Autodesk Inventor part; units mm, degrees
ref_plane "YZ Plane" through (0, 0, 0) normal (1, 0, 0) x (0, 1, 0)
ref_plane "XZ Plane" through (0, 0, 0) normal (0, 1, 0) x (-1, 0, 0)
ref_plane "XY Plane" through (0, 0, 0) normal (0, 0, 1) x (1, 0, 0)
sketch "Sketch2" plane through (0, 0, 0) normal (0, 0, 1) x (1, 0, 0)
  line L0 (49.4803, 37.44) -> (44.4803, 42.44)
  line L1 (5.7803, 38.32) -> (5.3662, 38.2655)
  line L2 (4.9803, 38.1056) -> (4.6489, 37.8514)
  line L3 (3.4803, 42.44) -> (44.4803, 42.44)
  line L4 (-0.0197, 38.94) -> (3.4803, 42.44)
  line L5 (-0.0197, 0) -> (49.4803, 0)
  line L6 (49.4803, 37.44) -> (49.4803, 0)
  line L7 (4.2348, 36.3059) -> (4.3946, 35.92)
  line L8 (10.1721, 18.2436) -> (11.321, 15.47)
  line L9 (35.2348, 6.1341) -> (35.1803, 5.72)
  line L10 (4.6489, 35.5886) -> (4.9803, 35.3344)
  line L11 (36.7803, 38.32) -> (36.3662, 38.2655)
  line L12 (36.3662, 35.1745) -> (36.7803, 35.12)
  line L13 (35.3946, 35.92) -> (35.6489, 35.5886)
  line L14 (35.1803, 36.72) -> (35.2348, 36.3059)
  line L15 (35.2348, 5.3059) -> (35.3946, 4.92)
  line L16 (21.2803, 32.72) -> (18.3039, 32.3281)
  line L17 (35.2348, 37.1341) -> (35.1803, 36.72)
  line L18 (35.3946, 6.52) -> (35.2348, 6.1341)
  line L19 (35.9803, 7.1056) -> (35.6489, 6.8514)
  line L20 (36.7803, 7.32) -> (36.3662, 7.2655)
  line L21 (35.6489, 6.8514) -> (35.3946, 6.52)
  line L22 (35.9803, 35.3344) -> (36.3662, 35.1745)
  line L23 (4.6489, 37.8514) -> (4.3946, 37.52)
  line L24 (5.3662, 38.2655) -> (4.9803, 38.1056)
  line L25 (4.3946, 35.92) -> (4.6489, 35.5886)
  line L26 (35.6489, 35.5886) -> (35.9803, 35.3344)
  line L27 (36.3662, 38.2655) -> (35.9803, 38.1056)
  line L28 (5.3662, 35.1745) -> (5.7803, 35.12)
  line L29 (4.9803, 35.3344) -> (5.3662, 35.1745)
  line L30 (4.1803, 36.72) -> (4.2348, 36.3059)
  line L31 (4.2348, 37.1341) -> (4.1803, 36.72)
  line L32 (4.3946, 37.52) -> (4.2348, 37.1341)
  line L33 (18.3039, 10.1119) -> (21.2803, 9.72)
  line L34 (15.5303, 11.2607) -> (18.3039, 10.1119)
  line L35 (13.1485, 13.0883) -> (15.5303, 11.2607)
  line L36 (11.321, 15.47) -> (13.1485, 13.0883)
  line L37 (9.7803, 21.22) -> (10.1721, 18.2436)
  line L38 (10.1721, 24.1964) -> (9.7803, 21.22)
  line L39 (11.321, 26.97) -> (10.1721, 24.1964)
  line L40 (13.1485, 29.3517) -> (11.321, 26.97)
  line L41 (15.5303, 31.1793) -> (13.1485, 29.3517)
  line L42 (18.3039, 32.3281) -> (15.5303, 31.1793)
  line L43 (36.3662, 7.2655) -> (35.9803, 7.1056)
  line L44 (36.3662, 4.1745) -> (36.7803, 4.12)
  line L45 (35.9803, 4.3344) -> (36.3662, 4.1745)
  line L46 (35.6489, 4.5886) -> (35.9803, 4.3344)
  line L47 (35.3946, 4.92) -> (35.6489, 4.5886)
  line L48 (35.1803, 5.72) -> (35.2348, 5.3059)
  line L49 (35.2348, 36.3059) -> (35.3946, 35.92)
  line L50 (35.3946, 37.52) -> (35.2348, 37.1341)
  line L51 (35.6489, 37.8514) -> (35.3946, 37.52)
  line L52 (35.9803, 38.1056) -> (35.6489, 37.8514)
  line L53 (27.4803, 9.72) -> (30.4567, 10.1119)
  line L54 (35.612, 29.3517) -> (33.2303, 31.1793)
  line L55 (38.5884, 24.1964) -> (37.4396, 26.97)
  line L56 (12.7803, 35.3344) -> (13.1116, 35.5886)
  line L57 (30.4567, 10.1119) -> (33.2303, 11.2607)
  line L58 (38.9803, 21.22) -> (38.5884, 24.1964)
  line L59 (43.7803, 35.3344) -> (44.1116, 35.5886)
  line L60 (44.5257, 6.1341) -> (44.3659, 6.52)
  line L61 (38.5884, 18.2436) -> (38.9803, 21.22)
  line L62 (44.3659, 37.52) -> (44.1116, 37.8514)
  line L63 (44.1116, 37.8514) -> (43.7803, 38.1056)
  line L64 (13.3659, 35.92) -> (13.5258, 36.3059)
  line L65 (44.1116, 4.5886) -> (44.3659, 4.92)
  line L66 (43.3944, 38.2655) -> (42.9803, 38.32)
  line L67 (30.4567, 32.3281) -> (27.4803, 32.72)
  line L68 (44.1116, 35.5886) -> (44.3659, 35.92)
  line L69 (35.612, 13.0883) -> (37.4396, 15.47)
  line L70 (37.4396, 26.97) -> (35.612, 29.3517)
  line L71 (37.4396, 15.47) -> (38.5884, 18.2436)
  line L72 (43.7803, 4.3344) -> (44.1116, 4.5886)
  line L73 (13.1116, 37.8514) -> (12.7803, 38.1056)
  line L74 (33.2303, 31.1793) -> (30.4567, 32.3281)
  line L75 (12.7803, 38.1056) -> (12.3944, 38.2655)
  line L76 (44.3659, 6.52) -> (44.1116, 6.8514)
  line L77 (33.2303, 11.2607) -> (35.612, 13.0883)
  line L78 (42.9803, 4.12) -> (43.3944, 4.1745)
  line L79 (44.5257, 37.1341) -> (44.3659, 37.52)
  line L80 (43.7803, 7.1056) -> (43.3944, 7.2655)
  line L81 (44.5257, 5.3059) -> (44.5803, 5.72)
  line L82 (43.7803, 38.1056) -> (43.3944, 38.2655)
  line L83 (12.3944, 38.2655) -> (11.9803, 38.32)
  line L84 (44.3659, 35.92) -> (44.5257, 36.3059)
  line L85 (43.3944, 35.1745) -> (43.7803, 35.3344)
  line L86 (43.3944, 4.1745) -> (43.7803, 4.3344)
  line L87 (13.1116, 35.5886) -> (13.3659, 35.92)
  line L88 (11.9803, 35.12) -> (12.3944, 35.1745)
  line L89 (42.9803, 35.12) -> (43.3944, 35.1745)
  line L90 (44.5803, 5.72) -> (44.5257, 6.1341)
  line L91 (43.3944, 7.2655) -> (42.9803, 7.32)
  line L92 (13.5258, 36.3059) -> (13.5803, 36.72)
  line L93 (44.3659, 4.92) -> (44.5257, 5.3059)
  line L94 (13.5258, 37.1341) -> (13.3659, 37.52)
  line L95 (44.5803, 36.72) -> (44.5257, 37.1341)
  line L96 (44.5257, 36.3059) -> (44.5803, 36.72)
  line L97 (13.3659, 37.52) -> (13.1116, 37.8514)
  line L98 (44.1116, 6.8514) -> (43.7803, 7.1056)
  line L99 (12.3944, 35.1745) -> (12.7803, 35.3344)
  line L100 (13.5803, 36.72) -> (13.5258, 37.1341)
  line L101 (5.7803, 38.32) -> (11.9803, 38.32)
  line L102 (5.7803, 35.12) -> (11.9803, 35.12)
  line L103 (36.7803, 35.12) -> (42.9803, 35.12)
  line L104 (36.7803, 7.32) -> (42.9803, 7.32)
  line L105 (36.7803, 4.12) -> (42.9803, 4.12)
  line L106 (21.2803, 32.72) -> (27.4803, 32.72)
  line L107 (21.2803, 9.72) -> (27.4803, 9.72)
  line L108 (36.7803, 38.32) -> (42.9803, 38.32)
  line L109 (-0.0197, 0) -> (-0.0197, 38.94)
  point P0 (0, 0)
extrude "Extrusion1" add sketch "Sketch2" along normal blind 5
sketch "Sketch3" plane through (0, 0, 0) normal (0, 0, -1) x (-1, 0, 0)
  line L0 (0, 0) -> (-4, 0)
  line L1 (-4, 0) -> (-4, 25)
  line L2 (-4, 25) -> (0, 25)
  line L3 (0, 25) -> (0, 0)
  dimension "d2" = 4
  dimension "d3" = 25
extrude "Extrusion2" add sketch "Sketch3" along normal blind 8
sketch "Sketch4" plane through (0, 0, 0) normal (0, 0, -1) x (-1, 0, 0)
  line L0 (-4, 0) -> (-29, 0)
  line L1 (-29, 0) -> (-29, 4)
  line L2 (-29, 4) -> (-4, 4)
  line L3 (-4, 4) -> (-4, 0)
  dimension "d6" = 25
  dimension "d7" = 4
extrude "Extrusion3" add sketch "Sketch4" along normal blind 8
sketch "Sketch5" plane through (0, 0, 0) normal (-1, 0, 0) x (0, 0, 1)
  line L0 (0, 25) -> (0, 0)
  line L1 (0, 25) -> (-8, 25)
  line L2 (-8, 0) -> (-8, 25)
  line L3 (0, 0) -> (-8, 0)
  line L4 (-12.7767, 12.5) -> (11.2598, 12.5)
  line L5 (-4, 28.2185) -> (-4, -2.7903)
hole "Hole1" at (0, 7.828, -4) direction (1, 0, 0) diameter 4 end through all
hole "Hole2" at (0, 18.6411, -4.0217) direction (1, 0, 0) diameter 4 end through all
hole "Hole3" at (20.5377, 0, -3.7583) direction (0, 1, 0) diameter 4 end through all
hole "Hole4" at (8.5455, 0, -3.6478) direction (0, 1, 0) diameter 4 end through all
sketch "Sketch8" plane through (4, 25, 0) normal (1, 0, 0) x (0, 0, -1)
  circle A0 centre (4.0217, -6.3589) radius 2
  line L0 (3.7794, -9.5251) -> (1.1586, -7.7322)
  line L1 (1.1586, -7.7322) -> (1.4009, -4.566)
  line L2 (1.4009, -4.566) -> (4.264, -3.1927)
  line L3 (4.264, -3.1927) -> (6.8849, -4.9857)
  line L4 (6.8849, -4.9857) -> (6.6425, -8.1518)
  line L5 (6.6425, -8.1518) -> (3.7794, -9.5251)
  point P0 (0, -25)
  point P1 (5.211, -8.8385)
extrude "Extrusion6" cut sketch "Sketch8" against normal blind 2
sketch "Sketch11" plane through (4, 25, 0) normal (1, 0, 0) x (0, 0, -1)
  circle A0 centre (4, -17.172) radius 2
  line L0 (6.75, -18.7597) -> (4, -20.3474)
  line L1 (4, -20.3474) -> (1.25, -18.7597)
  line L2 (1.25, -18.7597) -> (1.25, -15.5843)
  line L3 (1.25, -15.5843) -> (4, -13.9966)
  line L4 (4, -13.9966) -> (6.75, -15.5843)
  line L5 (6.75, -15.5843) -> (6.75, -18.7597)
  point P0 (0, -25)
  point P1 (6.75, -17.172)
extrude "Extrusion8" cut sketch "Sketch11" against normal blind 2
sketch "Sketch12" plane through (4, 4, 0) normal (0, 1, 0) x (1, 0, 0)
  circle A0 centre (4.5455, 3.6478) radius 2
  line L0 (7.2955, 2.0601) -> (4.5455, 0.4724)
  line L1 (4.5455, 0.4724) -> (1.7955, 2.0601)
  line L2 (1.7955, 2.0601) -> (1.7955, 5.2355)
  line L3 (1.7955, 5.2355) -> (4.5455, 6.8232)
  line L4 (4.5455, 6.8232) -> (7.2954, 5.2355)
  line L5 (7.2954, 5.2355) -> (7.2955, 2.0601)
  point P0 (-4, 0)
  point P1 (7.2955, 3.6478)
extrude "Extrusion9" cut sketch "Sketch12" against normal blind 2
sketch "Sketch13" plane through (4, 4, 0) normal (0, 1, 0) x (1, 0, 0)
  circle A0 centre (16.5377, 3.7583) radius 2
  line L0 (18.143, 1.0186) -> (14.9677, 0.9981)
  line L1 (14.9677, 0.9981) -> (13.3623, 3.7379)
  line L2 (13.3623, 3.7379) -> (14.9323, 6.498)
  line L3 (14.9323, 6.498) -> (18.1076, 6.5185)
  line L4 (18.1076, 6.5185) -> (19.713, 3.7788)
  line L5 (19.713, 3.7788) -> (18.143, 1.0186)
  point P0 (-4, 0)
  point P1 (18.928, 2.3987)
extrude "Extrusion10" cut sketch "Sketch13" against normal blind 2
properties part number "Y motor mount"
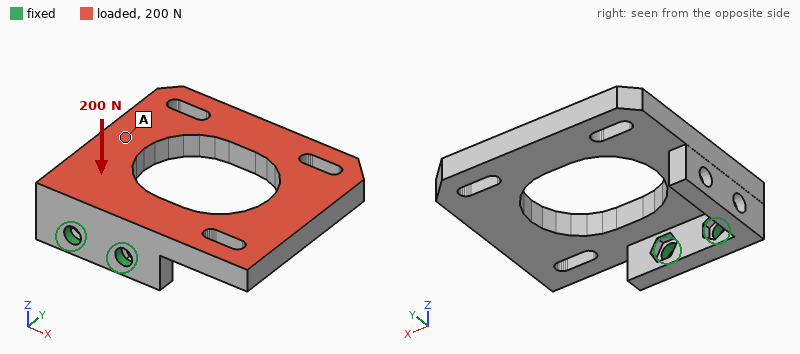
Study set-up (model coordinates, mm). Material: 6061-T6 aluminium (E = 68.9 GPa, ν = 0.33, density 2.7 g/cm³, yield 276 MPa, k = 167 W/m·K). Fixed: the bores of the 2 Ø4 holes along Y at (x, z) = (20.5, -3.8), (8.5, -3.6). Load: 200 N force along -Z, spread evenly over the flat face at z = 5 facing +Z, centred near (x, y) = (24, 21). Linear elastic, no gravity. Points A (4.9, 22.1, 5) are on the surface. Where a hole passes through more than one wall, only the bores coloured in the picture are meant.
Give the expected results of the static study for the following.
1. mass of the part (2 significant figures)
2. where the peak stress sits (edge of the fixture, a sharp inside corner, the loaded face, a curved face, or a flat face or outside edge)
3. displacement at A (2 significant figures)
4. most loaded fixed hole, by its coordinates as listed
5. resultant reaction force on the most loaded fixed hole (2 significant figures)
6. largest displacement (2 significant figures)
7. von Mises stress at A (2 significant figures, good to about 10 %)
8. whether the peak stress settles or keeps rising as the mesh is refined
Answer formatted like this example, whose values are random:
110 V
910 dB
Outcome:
23 g
edge of the fixture
0.068 mm
(20.5, -3.8)
250 N
0.25 mm
23 MPa
keeps rising
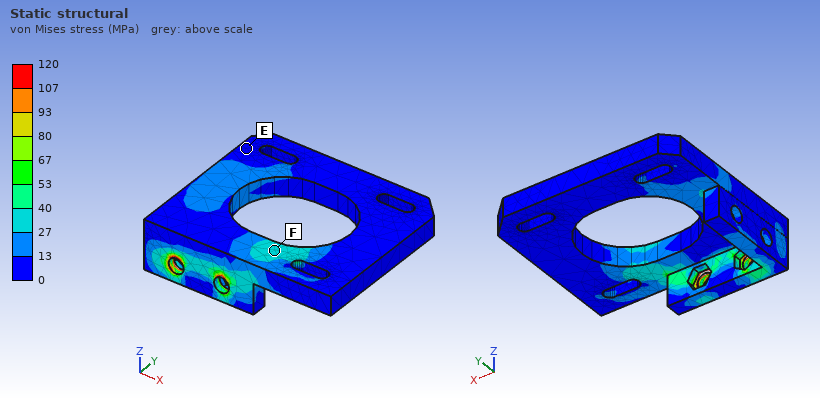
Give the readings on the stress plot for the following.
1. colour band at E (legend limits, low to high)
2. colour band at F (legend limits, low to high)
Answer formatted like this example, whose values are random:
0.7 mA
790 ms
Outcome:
0 to 13 MPa
27 to 40 MPa
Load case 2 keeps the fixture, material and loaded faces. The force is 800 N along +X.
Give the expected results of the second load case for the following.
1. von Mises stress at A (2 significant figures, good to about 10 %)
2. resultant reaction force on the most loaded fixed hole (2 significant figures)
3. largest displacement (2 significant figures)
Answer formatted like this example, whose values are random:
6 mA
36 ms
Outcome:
17 MPa
1.3 kN
0.15 mm
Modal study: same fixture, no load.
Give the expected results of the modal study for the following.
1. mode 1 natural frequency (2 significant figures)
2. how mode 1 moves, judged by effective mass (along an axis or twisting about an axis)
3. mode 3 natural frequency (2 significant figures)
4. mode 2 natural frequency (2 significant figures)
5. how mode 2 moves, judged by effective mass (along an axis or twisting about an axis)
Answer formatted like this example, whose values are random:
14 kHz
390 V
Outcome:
1300 Hz
along Z
3300 Hz
2400 Hz
along X
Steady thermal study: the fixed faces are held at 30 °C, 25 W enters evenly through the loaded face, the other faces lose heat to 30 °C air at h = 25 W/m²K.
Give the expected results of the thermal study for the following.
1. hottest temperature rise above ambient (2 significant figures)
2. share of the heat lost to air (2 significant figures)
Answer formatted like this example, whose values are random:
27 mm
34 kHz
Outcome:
36 K
8.4 %
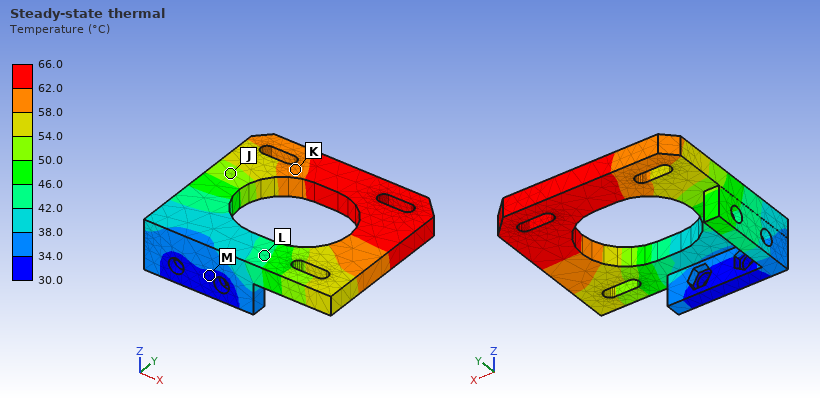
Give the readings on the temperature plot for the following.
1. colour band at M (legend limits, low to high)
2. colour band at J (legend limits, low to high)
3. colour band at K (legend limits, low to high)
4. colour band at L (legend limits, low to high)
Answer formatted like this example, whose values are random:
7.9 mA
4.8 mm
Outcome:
30.0 to 34.0 °C
50.0 to 54.0 °C
58.0 to 62.0 °C
42.0 to 46.0 °C
